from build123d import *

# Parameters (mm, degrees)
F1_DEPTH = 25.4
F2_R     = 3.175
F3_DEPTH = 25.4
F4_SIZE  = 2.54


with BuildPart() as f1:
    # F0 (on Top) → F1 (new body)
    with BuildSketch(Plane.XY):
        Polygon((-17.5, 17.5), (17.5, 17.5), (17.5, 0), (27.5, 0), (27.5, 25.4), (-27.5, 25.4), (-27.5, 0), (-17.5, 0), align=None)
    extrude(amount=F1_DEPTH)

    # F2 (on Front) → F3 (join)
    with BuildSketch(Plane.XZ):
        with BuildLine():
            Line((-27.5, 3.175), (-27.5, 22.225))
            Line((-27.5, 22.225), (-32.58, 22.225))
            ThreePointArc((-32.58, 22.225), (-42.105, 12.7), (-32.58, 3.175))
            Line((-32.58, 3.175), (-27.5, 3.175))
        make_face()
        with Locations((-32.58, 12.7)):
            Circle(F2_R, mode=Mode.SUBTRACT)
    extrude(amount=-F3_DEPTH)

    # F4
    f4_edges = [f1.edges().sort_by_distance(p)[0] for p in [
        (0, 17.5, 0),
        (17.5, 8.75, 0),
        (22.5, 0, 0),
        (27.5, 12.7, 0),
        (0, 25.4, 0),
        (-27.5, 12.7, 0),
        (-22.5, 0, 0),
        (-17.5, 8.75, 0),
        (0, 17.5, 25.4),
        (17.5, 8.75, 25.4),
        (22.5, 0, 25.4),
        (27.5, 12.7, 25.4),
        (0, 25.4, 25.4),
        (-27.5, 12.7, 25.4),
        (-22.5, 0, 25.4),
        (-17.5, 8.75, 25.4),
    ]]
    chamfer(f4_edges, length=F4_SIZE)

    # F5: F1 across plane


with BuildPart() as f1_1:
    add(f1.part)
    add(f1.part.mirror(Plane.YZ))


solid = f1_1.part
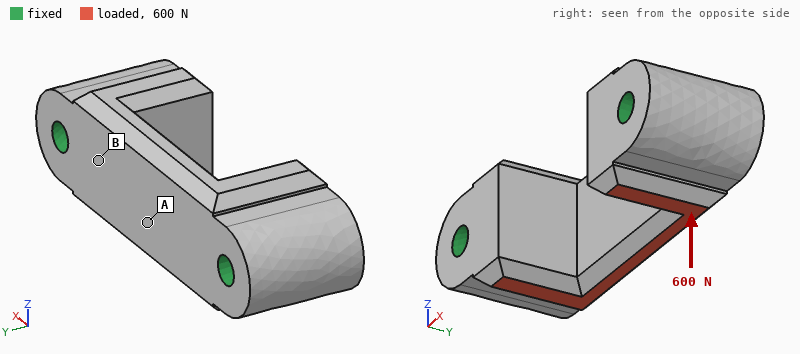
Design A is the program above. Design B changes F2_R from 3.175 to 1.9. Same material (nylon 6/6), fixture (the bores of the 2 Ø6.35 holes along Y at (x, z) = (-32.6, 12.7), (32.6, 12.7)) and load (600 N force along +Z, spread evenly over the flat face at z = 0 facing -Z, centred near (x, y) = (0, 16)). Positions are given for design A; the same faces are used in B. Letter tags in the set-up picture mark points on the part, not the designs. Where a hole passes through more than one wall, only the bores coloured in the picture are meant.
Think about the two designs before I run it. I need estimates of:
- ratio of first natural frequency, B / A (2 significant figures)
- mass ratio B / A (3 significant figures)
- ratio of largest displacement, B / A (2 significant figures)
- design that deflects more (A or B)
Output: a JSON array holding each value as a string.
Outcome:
["0.80", "1.04", "1.5", "B"]
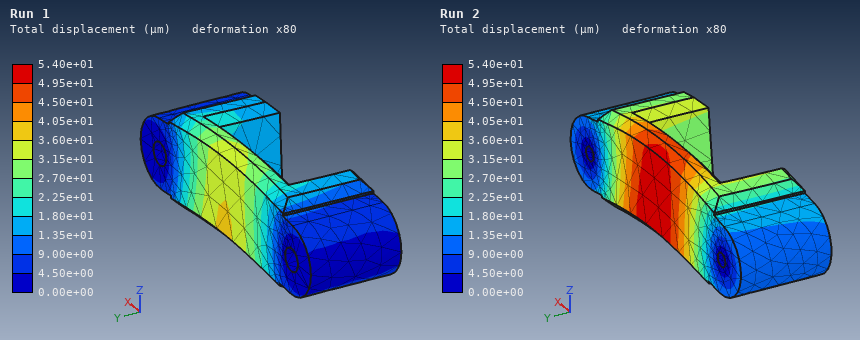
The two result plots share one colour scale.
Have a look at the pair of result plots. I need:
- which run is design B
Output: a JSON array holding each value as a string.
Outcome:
["Run 2"]
